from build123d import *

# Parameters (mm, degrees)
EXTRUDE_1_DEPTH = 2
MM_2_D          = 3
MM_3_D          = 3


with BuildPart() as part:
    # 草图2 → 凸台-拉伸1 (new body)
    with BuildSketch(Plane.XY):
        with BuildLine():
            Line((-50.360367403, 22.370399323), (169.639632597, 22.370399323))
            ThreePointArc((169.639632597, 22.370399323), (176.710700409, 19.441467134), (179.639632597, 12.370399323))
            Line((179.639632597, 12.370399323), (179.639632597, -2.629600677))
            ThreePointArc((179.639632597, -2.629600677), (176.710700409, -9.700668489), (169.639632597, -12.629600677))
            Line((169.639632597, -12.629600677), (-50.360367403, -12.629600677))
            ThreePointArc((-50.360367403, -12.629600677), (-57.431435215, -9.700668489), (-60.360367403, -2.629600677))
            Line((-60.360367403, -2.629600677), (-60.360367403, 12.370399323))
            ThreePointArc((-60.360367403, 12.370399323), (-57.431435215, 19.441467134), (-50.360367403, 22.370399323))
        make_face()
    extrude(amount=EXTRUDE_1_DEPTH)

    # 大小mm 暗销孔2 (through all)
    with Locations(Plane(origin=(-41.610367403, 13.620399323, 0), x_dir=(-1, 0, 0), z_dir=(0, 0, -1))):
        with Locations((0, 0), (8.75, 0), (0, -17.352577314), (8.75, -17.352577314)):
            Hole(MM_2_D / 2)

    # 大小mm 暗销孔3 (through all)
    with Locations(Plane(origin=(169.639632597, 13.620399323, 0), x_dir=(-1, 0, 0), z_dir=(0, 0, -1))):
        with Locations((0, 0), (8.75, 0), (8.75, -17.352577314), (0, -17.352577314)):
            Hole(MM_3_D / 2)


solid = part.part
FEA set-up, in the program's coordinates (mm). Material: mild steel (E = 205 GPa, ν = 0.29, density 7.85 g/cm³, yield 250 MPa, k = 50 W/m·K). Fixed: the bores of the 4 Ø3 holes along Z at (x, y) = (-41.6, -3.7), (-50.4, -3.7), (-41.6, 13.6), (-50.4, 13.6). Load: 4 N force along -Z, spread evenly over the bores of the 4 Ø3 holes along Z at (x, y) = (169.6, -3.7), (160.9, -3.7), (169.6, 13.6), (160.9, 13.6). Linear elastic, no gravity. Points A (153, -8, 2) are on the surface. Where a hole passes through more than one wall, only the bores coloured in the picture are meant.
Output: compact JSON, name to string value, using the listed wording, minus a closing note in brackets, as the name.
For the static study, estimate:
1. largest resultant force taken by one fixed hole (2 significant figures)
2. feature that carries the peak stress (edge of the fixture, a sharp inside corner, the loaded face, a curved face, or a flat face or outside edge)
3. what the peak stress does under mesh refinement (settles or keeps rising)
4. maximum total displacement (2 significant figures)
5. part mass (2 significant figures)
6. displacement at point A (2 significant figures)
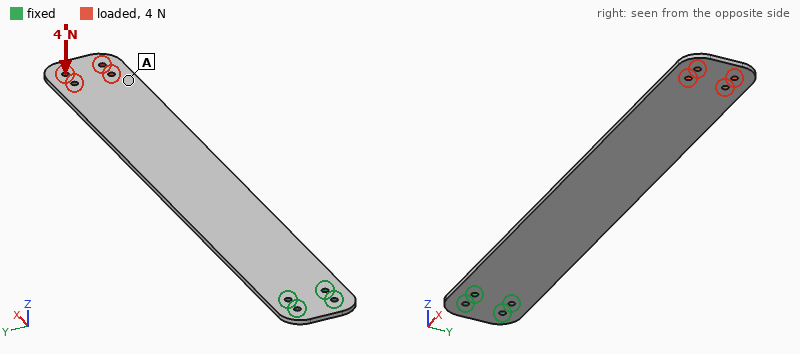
{"largest resultant force taken by one fixed hole": "17 N", "feature that carries the peak stress": "edge of the fixture", "what the peak stress does under mesh refinement": "keeps rising", "maximum total displacement": "2.7 mm", "part mass": "130 g", "displacement at point A": "2.2 mm"}
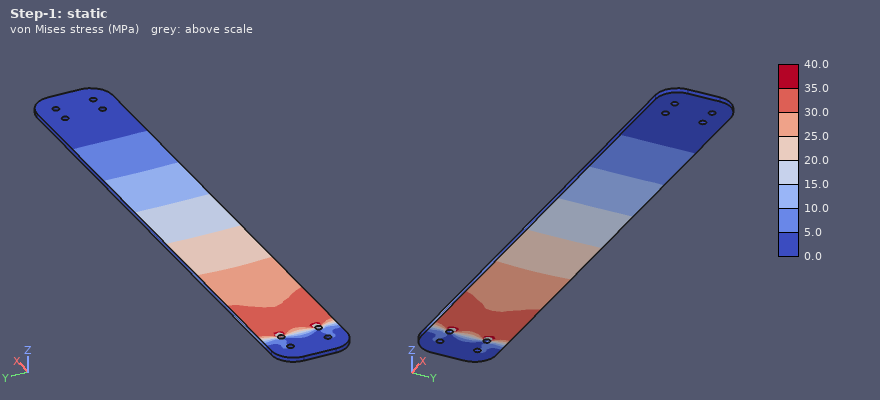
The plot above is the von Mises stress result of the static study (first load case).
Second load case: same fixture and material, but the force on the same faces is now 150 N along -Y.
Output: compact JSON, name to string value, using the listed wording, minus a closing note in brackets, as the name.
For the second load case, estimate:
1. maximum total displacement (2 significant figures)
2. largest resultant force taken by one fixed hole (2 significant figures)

{"maximum total displacement": "0.36 mm", "largest resultant force taken by one fixed hole": "1.1 kN"}
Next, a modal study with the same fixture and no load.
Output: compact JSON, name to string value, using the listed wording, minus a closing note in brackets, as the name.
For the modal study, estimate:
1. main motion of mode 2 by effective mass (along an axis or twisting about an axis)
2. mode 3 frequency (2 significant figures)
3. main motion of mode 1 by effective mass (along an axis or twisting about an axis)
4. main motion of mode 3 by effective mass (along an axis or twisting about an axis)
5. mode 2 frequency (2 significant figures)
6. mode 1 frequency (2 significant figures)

{"main motion of mode 2 by effective mass": "along Z", "mode 3 frequency": "430 Hz", "main motion of mode 1 by effective mass": "along Z", "main motion of mode 3 by effective mass": "twisting about X", "mode 2 frequency": "220 Hz", "mode 1 frequency": "35 Hz"}
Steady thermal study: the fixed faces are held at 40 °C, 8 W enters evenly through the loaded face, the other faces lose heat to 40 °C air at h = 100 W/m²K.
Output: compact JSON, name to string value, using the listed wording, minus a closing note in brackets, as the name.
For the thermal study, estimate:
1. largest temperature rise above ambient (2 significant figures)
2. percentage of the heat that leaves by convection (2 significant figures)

{"largest temperature rise above ambient": "33 K", "percentage of the heat that leaves by convection": "100 %"}
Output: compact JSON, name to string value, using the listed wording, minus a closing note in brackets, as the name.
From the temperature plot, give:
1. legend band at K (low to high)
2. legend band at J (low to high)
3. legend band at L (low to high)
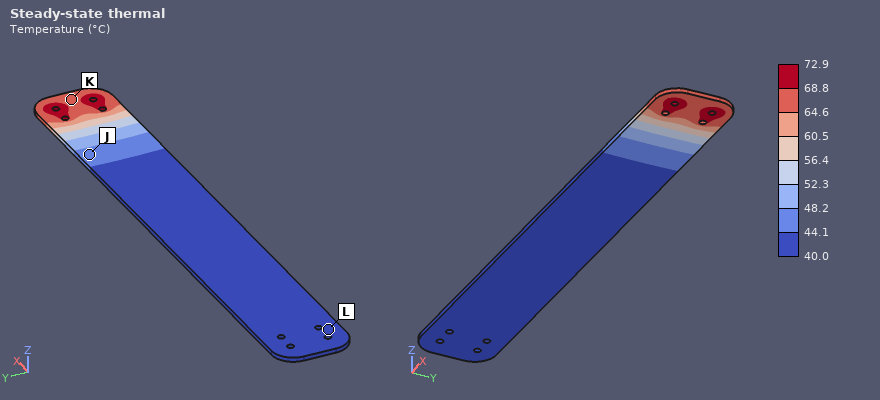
{"legend band at K": "64.6 to 68.8 °C", "legend band at J": "44.1 to 48.2 °C", "legend band at L": "40.0 to 44.1 °C"}
